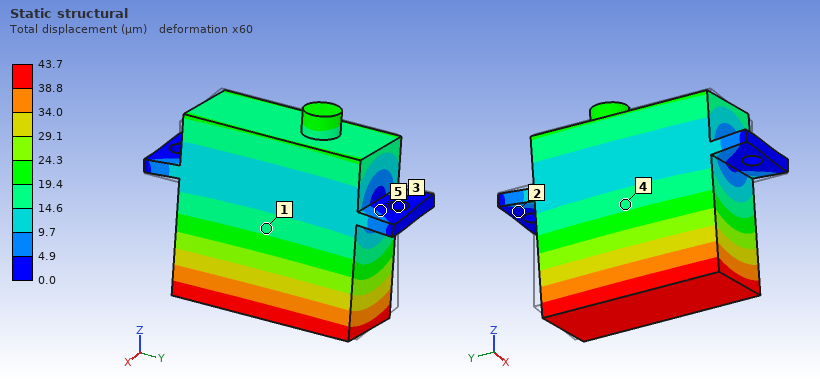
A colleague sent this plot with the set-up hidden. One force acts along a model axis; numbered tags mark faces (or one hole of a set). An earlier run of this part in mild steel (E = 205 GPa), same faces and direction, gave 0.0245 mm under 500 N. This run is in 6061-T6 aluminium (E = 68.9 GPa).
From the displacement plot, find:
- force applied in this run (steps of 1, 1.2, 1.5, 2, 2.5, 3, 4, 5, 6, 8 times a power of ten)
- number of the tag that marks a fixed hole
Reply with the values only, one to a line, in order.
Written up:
300 N
3
